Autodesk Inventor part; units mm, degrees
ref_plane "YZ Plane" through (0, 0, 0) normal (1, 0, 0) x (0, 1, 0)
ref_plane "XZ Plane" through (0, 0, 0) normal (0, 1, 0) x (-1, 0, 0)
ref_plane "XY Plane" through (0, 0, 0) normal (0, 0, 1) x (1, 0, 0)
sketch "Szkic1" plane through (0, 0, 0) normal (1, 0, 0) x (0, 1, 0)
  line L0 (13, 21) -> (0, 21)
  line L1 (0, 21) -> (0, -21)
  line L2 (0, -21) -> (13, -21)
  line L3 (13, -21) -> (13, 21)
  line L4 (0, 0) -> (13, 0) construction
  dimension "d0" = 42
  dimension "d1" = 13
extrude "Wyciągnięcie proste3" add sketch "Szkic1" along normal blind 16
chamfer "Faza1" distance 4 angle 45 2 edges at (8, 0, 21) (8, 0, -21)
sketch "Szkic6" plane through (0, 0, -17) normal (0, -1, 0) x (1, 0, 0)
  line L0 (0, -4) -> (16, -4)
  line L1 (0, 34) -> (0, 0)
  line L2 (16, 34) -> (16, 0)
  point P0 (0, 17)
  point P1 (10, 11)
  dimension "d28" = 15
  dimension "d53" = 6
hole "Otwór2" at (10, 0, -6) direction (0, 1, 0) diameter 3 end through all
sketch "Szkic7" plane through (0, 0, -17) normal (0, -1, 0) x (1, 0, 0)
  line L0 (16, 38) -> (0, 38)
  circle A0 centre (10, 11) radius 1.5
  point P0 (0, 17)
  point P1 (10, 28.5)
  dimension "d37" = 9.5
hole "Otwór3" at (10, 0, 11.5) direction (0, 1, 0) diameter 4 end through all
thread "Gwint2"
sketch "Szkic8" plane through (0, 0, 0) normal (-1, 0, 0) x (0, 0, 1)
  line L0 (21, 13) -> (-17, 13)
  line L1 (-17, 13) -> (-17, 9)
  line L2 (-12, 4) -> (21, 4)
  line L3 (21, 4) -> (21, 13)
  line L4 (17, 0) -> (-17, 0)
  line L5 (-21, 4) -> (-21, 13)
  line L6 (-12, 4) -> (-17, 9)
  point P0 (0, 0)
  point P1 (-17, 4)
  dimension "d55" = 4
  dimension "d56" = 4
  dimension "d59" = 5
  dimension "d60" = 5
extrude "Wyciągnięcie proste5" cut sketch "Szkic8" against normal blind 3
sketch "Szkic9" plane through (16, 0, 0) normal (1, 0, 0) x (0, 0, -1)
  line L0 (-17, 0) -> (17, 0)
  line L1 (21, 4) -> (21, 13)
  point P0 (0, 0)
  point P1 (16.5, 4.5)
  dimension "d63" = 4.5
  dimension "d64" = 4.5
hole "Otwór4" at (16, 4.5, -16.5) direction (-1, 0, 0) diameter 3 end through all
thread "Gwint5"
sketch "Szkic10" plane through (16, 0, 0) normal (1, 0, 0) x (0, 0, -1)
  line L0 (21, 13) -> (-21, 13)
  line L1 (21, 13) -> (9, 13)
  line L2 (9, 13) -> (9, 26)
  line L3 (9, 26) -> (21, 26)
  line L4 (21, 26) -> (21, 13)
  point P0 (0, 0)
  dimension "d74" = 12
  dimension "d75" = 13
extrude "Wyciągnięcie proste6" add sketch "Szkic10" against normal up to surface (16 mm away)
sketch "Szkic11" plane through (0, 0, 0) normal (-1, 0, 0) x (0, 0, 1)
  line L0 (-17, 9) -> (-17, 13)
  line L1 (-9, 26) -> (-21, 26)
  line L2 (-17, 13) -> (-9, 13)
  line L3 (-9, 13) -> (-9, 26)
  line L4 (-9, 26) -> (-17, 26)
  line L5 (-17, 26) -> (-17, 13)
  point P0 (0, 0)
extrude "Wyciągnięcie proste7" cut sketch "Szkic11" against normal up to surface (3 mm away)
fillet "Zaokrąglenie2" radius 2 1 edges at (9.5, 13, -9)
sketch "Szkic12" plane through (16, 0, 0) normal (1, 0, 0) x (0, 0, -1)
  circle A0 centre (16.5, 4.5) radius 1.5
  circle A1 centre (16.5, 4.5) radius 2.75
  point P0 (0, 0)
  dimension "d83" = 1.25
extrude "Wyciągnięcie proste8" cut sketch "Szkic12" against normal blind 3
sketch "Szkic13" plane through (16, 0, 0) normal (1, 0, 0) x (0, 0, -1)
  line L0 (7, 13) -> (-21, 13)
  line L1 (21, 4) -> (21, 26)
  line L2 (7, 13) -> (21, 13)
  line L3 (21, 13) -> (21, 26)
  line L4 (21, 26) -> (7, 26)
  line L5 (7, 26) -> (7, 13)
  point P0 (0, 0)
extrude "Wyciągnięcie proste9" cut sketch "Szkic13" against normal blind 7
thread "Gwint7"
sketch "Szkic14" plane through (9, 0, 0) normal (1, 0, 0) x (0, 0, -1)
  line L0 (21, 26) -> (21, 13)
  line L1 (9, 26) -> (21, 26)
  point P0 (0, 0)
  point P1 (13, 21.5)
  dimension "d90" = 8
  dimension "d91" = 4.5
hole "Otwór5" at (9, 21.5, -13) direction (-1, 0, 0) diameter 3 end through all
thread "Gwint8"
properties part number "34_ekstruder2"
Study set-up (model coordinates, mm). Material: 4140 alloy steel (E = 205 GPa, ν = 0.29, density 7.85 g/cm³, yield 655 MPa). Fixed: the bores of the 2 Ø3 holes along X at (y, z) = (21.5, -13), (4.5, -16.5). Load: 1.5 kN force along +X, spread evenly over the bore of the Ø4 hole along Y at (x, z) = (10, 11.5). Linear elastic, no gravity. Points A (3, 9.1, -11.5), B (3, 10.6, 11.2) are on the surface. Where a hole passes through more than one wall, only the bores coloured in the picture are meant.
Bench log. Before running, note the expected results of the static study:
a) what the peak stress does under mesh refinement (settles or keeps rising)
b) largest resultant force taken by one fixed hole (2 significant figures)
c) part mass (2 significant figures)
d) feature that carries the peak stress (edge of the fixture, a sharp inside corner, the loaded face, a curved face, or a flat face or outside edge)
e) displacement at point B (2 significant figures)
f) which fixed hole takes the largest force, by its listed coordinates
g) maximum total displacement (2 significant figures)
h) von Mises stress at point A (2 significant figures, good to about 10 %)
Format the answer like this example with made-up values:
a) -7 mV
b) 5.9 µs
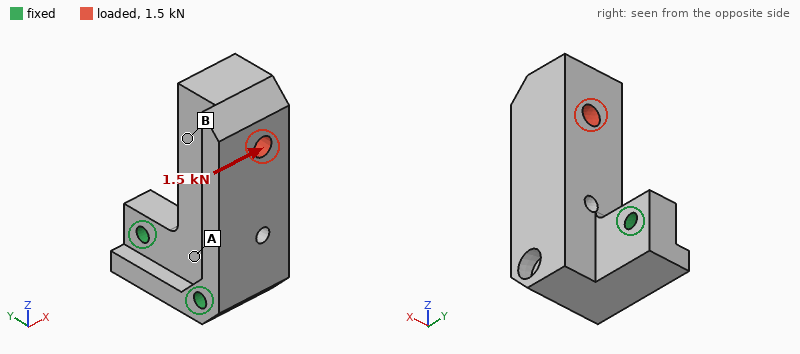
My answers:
a) keeps rising
b) 1.2 kN
c) 64 g
d) edge of the fixture
e) 30 µm
f) (4.5, -16.5)
g) 43 µm
h) 74 MPa
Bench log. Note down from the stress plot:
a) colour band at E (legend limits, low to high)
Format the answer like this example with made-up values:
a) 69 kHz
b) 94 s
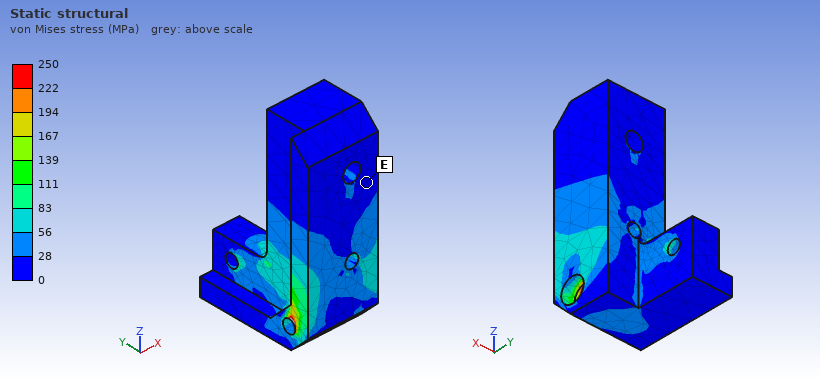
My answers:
a) 0 to 28 MPa
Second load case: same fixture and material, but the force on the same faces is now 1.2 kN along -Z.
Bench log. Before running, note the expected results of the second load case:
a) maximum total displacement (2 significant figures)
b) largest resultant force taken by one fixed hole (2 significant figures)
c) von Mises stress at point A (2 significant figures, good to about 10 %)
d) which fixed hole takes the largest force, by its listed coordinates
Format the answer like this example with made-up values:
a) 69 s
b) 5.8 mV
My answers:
a) 3.6 µm
b) 1.1 kN
c) 3.7 MPa
d) (4.5, -16.5)
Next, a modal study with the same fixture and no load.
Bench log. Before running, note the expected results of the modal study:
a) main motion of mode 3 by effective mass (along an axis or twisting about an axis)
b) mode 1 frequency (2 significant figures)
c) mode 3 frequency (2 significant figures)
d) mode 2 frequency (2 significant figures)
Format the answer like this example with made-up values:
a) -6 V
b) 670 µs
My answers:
a) twisting about Z
b) 6700 Hz
c) 18 kHz
d) 6800 Hz
